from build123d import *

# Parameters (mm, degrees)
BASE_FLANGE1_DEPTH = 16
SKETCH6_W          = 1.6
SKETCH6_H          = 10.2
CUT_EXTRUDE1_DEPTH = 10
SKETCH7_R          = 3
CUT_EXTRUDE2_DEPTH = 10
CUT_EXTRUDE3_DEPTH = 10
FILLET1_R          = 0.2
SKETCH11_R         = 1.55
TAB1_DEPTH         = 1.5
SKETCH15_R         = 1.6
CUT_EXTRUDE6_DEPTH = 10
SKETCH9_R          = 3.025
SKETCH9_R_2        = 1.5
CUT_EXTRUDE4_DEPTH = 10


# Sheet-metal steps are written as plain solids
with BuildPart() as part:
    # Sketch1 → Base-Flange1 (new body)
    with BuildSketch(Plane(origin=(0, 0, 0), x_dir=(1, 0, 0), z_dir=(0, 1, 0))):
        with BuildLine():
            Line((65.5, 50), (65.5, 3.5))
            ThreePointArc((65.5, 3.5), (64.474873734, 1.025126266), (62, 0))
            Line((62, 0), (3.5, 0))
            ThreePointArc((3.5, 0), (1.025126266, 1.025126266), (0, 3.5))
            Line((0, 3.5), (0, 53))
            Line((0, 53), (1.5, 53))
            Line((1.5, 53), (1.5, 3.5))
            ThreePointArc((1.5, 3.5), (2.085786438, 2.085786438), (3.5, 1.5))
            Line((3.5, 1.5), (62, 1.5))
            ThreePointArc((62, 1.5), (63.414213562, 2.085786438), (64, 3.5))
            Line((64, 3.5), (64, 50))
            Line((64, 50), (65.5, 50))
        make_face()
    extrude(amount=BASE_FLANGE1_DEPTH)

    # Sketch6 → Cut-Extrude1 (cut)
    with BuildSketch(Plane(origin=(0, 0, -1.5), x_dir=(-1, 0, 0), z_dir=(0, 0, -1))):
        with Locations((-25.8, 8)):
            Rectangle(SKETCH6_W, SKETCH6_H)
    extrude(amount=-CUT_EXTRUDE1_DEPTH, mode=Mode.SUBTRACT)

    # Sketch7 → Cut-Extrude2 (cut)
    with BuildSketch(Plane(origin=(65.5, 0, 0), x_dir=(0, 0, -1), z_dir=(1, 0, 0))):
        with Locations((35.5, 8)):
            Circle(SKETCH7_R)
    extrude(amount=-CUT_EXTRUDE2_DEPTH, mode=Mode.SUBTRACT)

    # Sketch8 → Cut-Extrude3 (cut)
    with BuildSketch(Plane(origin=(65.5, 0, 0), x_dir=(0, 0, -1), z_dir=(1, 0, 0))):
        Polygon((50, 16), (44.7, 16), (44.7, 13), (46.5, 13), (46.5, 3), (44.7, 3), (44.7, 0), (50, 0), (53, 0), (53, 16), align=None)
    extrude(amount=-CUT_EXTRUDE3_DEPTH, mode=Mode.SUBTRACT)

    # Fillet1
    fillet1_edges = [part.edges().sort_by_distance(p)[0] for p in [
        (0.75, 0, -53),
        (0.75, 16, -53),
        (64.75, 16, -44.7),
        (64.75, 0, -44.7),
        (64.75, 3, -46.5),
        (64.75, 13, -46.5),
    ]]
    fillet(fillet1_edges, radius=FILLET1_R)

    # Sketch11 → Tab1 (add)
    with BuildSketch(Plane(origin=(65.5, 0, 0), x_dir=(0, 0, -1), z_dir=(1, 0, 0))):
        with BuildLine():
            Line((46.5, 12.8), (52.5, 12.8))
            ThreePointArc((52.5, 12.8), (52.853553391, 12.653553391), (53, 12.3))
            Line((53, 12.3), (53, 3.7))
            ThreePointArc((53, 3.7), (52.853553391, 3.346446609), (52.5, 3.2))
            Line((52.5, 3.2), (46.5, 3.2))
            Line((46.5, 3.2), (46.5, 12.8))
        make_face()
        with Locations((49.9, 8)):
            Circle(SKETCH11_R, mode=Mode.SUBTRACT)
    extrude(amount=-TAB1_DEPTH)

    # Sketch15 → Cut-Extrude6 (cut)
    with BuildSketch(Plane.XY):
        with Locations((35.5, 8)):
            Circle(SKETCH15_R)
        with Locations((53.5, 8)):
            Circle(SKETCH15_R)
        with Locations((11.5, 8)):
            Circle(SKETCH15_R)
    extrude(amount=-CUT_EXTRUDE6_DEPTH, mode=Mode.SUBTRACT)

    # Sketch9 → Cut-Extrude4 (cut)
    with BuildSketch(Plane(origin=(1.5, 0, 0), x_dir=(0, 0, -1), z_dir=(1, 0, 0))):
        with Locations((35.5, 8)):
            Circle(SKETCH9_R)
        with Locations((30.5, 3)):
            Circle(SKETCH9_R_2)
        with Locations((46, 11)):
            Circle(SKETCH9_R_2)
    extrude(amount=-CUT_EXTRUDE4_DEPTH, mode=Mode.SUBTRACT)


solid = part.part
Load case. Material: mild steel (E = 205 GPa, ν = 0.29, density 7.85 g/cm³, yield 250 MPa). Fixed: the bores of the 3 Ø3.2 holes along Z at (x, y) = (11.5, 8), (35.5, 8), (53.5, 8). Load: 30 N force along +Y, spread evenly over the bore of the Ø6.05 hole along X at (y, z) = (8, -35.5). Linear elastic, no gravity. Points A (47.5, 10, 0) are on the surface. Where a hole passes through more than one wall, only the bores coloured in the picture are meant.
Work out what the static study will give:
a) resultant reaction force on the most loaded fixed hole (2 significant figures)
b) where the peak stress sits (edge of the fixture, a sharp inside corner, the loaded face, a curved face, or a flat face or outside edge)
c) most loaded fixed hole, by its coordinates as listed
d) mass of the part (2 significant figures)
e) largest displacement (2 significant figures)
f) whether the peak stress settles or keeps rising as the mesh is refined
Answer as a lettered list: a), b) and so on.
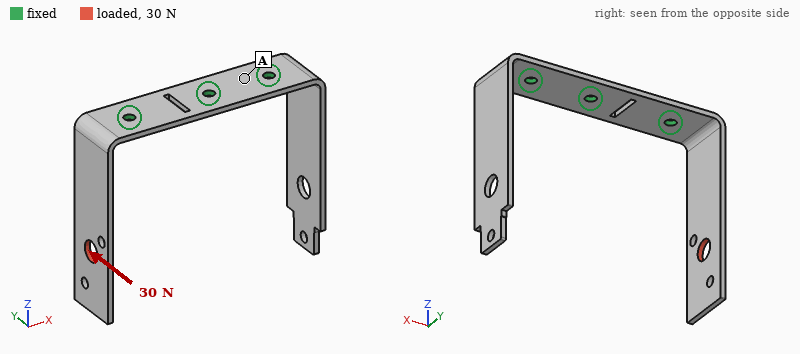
a) 38 N
b) edge of the fixture
c) (11.5, 8)
d) 29 g
e) 0.33 mm
f) keeps rising
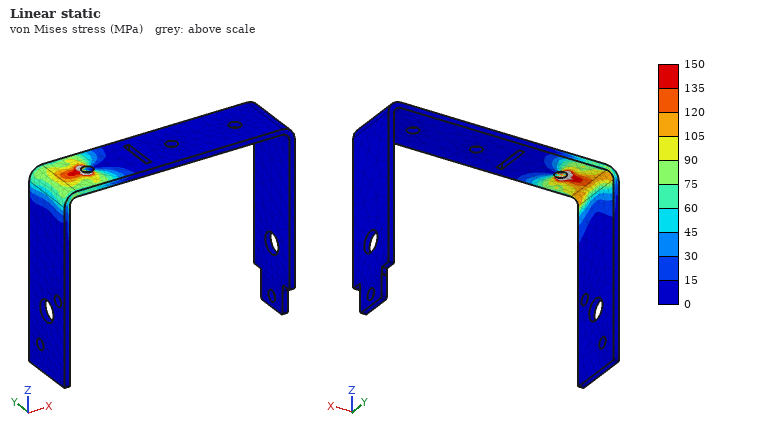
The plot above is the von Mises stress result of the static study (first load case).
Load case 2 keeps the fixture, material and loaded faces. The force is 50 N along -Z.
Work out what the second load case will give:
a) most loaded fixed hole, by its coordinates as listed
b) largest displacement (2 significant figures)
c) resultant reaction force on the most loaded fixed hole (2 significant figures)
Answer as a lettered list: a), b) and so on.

a) (11.5, 8)
b) 0.15 mm
c) 52 N
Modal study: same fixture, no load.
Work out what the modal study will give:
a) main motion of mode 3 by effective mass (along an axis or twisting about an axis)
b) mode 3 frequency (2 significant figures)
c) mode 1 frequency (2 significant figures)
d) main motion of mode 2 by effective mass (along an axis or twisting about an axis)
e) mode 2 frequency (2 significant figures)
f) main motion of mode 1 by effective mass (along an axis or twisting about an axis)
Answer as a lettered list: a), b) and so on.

a) along Y
b) 710 Hz
c) 360 Hz
d) along X
e) 400 Hz
f) along X
